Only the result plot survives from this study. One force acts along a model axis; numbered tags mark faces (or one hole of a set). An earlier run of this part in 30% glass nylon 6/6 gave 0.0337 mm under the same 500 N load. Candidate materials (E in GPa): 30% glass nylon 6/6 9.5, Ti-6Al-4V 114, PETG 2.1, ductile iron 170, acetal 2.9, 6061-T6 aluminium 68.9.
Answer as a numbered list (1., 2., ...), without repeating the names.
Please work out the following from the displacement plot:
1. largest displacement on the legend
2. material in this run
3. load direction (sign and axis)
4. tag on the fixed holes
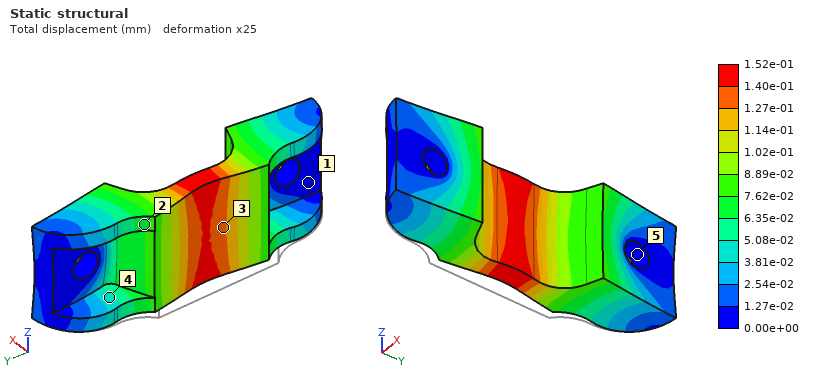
1. 1.52e-01 mm
2. PETG
3. +X
4. 5
